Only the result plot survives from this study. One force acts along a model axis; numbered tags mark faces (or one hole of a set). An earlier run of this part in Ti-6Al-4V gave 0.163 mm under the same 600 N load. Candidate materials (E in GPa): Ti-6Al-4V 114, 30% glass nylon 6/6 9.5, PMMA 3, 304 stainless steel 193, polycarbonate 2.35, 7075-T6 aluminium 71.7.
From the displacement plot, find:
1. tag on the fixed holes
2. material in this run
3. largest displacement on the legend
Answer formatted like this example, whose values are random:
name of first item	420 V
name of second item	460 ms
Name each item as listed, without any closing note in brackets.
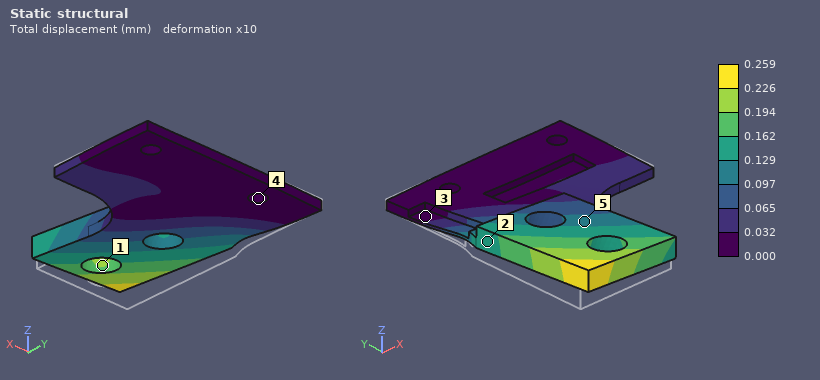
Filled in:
tag on the fixed holes	4
material in this run	7075-T6 aluminium
largest displacement on the legend	0.259 mm
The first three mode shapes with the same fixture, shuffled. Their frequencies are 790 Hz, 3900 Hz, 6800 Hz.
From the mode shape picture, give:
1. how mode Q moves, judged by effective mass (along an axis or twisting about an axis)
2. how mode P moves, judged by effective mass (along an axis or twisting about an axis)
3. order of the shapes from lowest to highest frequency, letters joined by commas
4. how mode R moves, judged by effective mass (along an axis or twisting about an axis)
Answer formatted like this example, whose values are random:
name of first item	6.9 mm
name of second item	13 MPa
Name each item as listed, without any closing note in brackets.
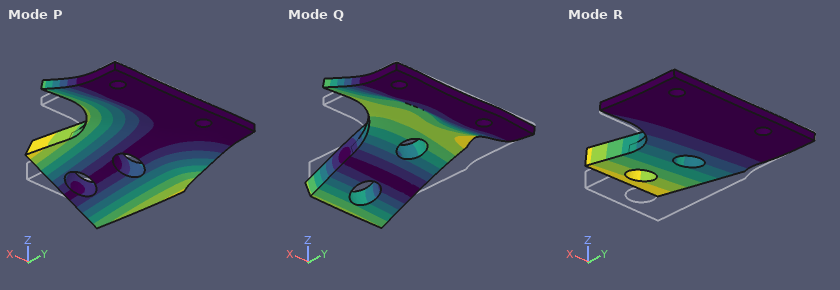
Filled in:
how mode Q moves, judged by effective mass	along Z
how mode P moves, judged by effective mass	twisting about Y
order of the shapes from lowest to highest frequency, letters joined by commas	R, P, Q
how mode R moves, judged by effective mass	along Z
